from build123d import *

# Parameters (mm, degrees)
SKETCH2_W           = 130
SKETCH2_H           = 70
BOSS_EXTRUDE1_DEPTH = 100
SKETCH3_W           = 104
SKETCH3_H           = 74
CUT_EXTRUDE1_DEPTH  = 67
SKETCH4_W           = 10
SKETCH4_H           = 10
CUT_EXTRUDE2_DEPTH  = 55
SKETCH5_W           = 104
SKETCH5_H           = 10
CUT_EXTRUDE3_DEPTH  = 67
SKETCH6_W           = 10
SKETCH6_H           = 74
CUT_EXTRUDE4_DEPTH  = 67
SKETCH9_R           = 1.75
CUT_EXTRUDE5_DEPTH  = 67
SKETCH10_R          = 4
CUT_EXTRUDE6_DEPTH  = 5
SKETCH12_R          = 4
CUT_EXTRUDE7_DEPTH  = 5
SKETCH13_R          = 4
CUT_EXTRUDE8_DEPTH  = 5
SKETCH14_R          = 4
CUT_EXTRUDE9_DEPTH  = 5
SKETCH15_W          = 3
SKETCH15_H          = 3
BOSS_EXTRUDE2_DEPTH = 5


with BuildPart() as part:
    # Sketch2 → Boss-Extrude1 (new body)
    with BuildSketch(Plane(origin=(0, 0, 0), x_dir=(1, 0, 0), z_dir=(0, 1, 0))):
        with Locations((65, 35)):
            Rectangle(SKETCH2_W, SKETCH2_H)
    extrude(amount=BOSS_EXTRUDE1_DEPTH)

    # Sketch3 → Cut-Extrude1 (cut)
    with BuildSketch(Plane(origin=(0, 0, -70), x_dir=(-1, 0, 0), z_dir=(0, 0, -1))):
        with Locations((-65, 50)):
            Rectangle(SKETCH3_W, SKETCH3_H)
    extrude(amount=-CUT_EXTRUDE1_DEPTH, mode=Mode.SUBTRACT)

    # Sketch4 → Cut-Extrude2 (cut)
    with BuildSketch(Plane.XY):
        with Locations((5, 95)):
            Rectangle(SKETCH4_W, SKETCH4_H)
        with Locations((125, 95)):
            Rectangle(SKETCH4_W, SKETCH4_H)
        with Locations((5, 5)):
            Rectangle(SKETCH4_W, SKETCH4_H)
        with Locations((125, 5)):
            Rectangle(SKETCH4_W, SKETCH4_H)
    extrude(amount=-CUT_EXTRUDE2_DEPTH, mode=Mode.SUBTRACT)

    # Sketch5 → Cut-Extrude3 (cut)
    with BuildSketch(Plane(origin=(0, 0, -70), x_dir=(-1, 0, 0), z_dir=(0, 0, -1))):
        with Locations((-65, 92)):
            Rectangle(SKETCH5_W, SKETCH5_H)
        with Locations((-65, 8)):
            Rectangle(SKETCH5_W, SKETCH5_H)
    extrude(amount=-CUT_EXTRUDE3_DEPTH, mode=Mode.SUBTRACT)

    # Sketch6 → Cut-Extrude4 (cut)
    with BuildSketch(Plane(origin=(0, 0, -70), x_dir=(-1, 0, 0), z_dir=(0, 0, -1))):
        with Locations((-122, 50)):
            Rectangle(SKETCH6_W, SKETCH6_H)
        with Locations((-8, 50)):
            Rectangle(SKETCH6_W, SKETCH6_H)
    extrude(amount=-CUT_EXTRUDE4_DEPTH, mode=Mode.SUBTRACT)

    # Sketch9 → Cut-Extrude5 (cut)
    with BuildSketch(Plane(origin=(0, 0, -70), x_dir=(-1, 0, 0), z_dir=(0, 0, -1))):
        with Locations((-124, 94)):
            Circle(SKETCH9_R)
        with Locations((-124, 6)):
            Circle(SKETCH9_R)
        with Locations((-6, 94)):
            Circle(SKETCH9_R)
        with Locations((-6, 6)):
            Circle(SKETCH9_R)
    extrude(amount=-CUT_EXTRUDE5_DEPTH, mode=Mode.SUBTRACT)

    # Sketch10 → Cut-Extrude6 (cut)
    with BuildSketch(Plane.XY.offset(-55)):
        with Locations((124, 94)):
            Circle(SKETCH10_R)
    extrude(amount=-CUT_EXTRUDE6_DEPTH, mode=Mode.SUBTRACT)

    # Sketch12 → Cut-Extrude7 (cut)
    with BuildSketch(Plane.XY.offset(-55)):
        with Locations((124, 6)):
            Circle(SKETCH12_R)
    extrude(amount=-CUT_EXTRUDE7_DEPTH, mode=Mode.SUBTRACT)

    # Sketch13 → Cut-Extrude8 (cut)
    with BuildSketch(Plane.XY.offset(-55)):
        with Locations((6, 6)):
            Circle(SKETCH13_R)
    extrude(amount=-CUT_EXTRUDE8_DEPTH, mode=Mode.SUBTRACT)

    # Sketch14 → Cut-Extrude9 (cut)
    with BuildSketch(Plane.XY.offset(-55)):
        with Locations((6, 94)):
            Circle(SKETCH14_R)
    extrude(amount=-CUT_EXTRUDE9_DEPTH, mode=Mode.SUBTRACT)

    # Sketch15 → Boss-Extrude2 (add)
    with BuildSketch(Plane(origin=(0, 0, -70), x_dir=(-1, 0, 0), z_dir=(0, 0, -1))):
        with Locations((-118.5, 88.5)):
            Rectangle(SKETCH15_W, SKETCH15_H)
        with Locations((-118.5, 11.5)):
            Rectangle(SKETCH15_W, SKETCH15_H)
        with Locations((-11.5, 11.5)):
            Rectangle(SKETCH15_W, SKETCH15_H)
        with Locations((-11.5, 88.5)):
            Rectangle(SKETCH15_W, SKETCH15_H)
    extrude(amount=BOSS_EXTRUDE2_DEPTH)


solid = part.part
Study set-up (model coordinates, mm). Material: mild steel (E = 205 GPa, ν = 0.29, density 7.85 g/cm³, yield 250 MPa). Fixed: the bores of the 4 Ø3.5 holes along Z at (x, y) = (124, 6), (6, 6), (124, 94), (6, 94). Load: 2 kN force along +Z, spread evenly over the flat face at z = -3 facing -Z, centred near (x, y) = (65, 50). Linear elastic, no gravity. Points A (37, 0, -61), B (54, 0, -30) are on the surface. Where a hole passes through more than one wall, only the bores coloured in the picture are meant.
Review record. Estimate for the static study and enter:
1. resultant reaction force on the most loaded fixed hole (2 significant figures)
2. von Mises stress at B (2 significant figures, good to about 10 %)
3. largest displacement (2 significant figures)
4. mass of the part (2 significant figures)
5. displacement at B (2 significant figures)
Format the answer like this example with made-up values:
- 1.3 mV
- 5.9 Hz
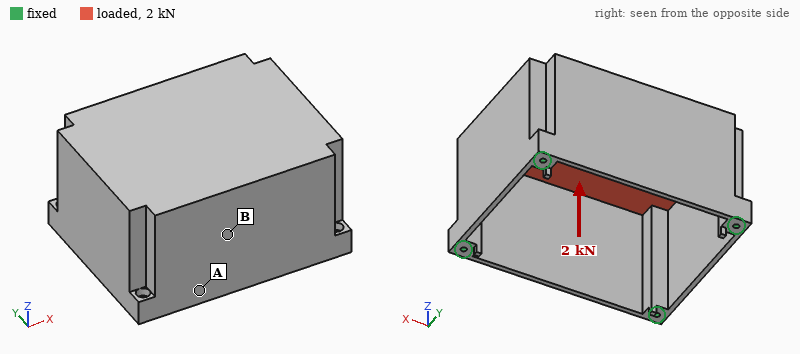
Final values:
- 520 N
- 9.6 MPa
- 92 µm
- 1.0 kg
- 19 µm
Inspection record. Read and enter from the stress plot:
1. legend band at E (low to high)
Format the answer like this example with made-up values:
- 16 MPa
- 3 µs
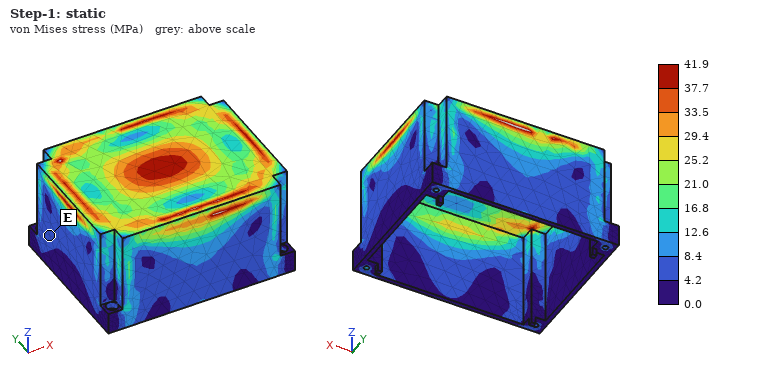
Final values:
- 4.2 to 8.4 MPa
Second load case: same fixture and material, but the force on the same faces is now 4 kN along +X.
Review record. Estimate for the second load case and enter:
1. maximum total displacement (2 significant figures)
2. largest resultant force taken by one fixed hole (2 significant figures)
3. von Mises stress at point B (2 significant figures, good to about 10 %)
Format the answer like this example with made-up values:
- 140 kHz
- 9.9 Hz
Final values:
- 9.8 µm
- 1.4 kN
- 12 MPa
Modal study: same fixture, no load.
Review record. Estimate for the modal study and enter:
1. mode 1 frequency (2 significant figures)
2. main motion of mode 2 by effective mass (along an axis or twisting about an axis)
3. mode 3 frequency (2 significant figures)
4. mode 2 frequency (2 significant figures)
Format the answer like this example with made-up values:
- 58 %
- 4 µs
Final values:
- 1500 Hz
- along Y
- 1900 Hz
- 1600 Hz
